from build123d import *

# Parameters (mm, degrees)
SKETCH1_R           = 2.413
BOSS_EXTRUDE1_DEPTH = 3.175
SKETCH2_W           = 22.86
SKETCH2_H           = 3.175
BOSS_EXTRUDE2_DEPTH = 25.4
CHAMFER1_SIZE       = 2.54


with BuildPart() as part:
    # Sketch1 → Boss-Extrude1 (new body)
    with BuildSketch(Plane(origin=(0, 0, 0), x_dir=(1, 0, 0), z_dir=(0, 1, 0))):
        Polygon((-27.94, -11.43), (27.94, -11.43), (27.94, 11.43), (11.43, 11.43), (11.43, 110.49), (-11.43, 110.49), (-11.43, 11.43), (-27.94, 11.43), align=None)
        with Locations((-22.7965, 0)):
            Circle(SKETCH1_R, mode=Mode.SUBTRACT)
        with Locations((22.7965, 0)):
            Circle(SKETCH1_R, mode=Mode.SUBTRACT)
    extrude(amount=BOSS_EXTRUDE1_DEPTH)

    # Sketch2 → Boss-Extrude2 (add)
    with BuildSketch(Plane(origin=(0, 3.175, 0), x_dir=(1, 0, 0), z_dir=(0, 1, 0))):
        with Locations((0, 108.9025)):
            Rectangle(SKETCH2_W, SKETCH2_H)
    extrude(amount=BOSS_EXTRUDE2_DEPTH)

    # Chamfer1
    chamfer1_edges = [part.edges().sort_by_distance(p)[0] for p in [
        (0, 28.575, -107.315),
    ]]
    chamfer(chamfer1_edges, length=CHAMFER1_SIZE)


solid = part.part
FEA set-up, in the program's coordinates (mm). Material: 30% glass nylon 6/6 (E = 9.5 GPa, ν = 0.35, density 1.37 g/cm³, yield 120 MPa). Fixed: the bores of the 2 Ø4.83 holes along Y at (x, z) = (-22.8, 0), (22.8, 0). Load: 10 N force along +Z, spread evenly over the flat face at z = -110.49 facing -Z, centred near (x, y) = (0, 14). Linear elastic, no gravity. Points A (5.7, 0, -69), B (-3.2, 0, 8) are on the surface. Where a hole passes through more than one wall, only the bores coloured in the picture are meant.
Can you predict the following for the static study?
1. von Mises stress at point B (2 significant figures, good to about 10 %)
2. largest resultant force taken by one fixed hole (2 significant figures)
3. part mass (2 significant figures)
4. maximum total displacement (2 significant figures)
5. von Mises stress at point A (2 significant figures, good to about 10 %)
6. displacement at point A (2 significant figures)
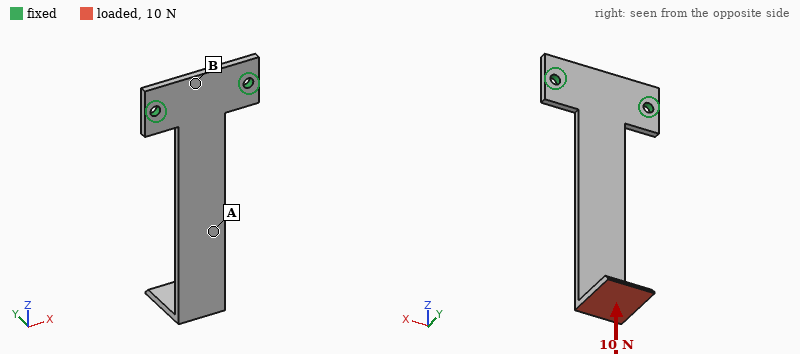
0.55 MPa
5.2 N
18 g
1.5 mm
3.2 MPa
0.52 mm
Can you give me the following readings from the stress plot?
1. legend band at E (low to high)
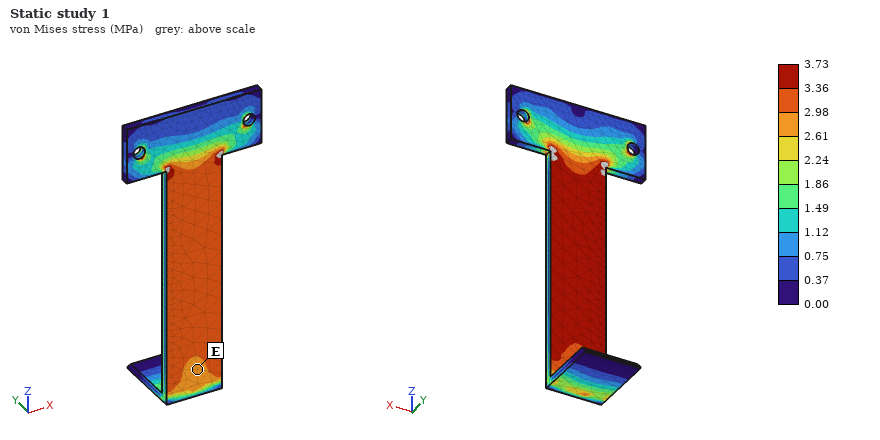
2.61 to 2.98 MPa
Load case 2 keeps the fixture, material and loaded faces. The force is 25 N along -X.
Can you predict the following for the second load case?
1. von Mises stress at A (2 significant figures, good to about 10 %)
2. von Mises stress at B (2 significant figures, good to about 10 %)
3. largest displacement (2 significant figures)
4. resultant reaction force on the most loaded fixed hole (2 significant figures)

7.4 MPa
1.7 MPa
1.5 mm
66 N
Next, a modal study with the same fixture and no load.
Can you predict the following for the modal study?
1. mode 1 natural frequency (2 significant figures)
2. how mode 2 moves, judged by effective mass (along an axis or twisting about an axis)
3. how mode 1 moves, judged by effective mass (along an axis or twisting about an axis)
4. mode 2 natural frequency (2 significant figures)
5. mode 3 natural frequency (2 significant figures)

81 Hz
along X
along Y
430 Hz
500 Hz
